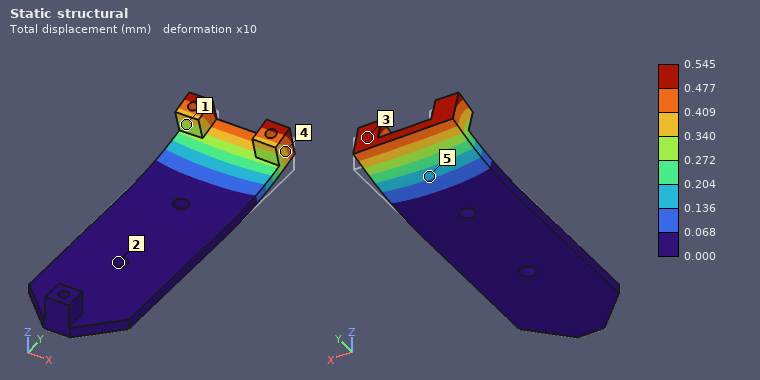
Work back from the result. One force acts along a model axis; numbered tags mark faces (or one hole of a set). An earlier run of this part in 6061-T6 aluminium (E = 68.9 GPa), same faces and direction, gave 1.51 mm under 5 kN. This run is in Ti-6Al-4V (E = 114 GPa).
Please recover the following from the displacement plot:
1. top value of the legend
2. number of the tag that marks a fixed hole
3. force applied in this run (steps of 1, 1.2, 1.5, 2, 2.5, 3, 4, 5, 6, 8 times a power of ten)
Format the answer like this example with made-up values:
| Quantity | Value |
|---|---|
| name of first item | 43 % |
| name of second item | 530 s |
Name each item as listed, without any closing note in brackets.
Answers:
| Quantity | Value |
|---|---|
| top value of the legend | 0.545 mm |
| number of the tag that marks a fixed hole | 2 |
| force applied in this run | 3 kN |
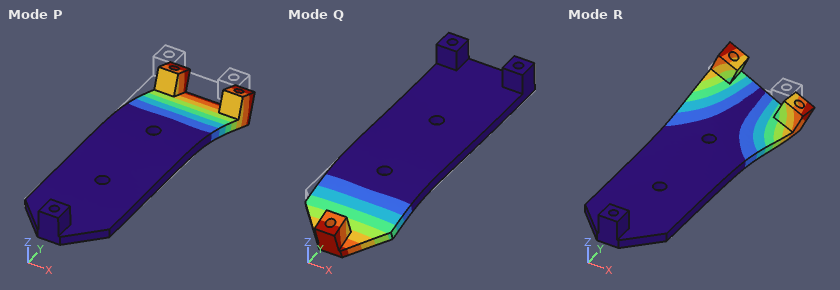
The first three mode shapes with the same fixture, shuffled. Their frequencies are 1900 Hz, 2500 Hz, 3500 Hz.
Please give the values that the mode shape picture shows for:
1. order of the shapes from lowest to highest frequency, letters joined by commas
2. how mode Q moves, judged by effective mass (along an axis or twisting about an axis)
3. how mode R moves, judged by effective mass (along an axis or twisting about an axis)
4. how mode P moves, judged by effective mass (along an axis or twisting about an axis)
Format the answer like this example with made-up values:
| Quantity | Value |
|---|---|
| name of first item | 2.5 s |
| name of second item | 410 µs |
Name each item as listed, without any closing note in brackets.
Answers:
| Quantity | Value |
|---|---|
| order of the shapes from lowest to highest frequency, letters joined by commas | P, Q, R |
| how mode Q moves, judged by effective mass | along Z |
| how mode R moves, judged by effective mass | twisting about Y |
| how mode P moves, judged by effective mass | along Z |
